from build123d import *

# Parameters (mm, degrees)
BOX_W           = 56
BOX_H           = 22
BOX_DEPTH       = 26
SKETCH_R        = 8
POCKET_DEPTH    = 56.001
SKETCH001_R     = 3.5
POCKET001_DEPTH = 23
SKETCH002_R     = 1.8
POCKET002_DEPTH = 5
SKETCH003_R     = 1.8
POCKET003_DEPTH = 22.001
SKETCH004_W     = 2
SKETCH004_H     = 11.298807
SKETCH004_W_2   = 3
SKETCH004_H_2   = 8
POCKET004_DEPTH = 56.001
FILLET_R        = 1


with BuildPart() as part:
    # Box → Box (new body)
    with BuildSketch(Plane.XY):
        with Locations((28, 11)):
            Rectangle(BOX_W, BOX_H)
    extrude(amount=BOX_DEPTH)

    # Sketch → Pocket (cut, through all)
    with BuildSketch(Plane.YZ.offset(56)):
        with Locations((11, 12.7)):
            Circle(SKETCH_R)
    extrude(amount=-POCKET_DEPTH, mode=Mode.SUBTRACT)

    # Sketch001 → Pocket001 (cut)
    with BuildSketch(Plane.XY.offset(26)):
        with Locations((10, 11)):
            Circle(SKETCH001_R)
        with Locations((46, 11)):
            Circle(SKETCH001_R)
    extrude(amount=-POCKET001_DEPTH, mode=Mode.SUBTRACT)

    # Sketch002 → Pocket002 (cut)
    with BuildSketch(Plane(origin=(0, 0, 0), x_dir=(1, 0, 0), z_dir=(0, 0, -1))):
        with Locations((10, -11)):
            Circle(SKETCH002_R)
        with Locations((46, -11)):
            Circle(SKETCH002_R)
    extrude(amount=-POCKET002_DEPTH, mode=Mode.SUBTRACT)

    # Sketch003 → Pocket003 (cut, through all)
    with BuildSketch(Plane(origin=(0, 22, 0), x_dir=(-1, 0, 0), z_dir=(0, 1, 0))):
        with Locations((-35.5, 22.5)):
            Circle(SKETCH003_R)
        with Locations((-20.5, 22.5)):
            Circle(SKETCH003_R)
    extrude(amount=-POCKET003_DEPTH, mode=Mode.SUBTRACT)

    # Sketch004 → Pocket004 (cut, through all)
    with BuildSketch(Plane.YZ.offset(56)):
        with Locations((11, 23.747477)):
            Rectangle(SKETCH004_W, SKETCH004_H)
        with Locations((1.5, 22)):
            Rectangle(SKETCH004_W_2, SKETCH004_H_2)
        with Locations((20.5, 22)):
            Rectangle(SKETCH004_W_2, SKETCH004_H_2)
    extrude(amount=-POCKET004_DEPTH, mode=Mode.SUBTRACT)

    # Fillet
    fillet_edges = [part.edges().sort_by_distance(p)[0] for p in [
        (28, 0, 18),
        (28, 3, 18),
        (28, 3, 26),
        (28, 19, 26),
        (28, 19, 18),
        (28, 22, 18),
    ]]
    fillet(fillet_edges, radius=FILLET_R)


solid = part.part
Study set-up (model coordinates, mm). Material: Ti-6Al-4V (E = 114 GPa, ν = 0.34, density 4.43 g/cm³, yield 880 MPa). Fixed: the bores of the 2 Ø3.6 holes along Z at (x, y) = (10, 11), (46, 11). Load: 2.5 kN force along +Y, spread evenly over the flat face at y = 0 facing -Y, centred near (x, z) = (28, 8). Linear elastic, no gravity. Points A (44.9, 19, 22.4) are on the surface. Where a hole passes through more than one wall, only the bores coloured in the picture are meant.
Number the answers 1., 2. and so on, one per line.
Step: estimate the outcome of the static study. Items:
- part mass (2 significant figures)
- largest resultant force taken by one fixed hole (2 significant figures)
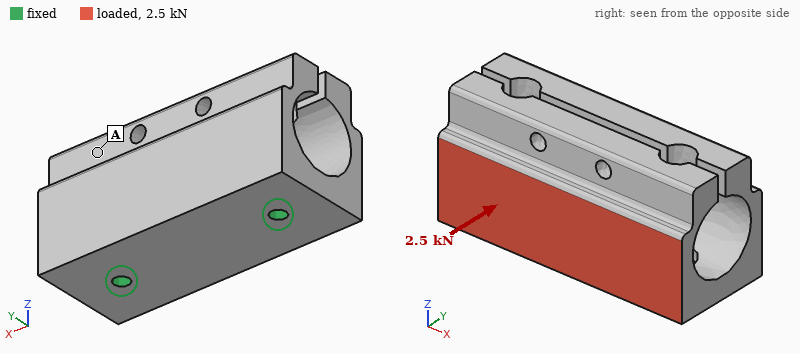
1. 74 g
2. 1.3 kN
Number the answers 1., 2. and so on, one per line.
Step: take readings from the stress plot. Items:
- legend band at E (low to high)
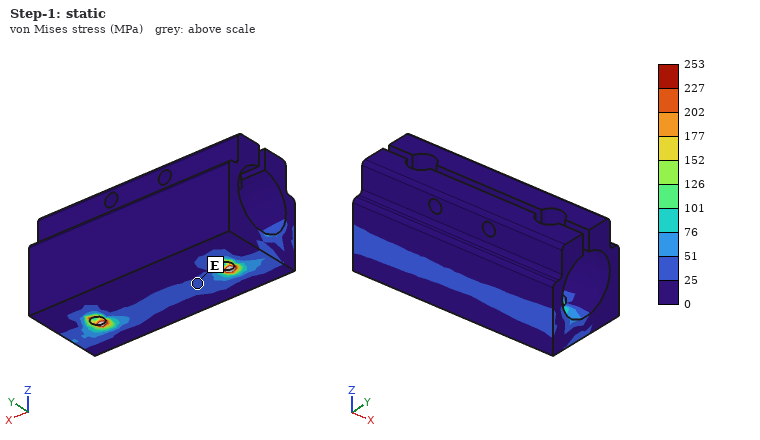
1. 25 to 51 MPa
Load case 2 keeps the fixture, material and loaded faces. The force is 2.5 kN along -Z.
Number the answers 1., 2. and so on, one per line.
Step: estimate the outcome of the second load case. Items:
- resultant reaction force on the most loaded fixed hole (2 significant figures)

1. 1.3 kN
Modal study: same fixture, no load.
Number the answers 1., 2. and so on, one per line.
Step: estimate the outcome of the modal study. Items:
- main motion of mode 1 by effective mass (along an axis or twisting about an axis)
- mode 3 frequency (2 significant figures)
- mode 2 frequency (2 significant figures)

1. along Y
2. 5400 Hz
3. 4300 Hz
